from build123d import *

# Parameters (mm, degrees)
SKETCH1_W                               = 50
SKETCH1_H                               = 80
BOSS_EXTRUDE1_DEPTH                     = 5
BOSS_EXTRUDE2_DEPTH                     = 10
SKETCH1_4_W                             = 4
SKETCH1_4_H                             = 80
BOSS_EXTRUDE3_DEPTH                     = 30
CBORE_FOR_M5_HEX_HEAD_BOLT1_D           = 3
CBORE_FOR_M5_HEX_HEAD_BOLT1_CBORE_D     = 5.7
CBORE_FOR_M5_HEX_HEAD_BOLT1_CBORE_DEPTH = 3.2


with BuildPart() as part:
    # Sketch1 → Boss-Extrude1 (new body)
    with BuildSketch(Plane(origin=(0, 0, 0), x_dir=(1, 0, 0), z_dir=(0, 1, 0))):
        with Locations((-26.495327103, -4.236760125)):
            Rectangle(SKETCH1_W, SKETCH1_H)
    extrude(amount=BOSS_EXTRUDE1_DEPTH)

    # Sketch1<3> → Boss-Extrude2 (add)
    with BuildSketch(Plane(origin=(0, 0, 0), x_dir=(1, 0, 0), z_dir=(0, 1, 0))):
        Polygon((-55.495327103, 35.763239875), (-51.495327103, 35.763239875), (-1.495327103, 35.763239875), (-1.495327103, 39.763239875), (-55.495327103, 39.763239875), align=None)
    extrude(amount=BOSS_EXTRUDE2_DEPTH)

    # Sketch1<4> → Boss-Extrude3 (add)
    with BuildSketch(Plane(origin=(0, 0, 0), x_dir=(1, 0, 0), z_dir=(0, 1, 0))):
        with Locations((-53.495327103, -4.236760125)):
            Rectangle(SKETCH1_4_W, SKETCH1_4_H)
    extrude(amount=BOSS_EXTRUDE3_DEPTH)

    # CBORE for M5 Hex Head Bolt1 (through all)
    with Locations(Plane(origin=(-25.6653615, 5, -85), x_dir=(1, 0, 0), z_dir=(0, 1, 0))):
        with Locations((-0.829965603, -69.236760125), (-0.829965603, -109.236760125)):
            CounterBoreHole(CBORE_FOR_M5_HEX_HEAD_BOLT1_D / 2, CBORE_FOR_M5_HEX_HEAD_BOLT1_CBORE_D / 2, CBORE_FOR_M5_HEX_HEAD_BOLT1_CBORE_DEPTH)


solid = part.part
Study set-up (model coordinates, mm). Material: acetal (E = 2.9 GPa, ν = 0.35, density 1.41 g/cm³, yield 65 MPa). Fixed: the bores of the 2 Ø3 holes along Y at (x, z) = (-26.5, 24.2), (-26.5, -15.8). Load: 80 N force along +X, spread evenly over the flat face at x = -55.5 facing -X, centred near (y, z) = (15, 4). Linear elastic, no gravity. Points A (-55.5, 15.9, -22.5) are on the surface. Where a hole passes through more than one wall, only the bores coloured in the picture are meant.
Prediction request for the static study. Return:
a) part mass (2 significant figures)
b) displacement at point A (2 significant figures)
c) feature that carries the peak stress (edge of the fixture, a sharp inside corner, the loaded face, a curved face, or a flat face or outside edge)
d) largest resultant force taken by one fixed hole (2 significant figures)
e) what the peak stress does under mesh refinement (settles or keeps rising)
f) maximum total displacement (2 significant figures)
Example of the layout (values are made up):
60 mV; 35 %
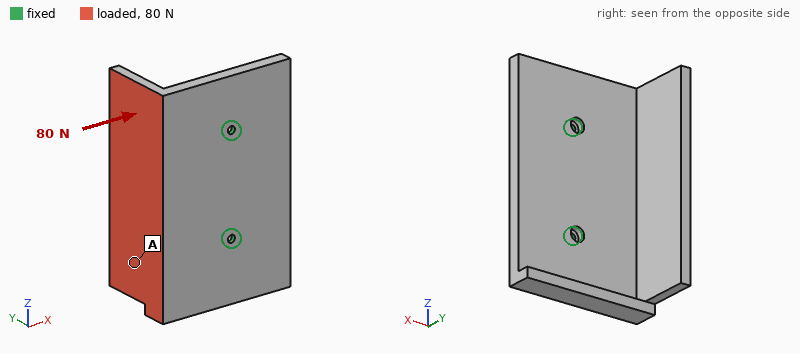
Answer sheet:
45 g; 0.85 mm; edge of the fixture; 41 N; keeps rising; 1.2 mm
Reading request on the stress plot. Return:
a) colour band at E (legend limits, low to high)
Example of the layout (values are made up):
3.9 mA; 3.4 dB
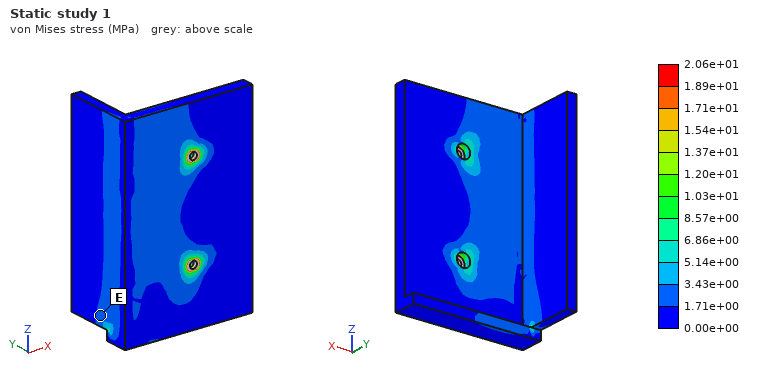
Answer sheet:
1.71e+00 to 3.43e+00 MPa
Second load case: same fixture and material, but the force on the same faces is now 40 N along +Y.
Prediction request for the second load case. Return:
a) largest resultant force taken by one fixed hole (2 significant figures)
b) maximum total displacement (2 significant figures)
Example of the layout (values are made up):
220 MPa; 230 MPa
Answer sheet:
21 N; 1.1 mm
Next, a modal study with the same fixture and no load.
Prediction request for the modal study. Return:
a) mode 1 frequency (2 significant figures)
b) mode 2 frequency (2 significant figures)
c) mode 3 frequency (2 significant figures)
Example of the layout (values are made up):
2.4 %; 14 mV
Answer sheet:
240 Hz; 610 Hz; 1100 Hz
